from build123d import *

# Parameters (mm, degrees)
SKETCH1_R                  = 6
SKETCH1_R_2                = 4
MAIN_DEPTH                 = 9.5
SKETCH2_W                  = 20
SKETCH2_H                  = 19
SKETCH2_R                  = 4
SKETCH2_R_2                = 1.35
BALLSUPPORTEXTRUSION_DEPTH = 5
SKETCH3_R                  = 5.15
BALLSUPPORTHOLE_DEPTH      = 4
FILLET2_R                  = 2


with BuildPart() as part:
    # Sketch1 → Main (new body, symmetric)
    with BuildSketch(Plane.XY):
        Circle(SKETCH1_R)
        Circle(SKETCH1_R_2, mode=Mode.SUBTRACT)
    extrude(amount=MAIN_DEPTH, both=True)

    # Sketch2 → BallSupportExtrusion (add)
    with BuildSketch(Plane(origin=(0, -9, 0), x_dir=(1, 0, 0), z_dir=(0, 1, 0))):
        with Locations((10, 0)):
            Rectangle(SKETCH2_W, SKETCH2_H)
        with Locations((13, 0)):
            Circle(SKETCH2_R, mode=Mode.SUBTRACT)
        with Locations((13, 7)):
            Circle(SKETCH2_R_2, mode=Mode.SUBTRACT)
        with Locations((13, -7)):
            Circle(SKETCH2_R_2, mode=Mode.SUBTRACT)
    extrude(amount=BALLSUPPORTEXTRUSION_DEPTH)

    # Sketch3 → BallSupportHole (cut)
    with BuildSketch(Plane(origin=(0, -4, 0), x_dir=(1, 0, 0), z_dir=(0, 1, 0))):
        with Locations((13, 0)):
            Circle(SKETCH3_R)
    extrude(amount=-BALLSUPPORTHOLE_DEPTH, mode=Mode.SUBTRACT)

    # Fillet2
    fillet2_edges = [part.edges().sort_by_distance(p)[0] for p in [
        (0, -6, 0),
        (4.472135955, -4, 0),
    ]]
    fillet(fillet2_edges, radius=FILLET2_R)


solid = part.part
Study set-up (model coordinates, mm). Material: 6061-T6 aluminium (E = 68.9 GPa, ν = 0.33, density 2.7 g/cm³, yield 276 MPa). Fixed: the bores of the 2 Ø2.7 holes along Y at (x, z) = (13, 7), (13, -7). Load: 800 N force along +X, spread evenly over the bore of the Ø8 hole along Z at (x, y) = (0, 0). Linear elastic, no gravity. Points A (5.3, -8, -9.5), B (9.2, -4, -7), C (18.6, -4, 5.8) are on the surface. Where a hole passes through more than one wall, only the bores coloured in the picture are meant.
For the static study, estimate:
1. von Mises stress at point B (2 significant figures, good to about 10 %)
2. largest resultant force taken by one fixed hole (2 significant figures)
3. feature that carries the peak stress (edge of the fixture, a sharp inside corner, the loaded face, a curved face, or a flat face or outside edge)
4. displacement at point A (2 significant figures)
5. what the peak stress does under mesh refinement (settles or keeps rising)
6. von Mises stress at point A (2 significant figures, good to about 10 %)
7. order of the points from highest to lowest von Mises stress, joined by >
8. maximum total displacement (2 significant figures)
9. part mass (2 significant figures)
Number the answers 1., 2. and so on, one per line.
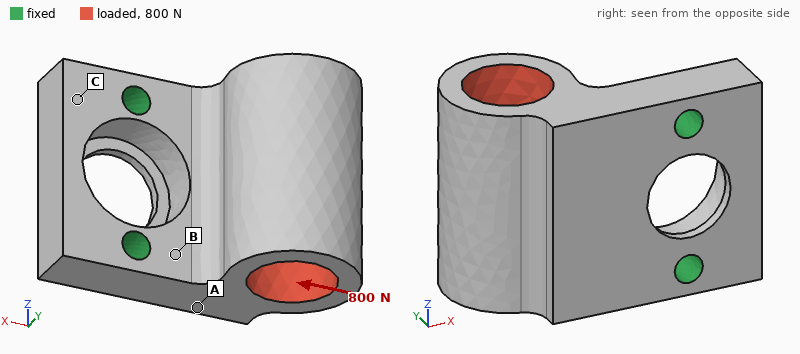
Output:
1. 130 MPa
2. 410 N
3. edge of the fixture
4. 16 µm
5. keeps rising
6. 35 MPa
7. B > A > C
8. 98 µm
9. 7.0 g
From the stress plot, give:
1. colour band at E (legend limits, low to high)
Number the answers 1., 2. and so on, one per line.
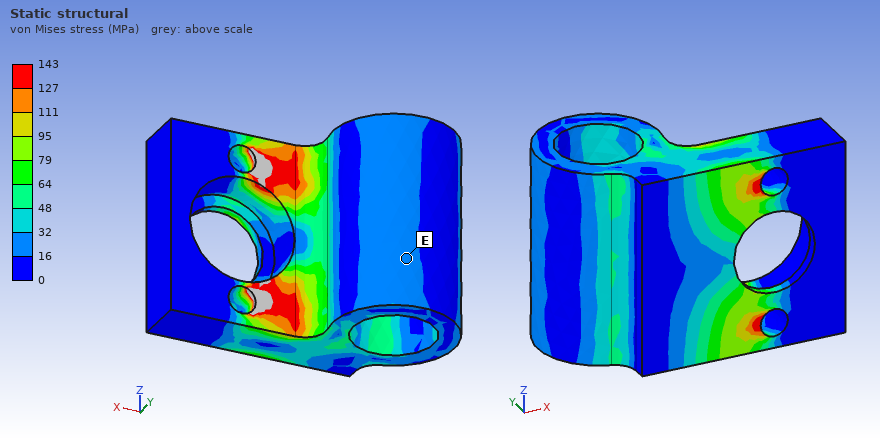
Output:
1. 16 to 32 MPa
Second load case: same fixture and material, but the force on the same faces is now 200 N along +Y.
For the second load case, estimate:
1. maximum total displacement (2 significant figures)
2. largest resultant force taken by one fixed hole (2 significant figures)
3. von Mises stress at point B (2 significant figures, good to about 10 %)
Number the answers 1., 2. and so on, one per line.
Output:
1. 31 µm
2. 100 N
3. 43 MPa
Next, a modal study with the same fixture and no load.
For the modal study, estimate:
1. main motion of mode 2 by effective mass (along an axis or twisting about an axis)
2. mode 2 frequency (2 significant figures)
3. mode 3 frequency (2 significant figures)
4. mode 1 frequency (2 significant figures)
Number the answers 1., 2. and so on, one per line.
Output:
1. along Z
2. 16 kHz
3. 24 kHz
4. 6800 Hz
